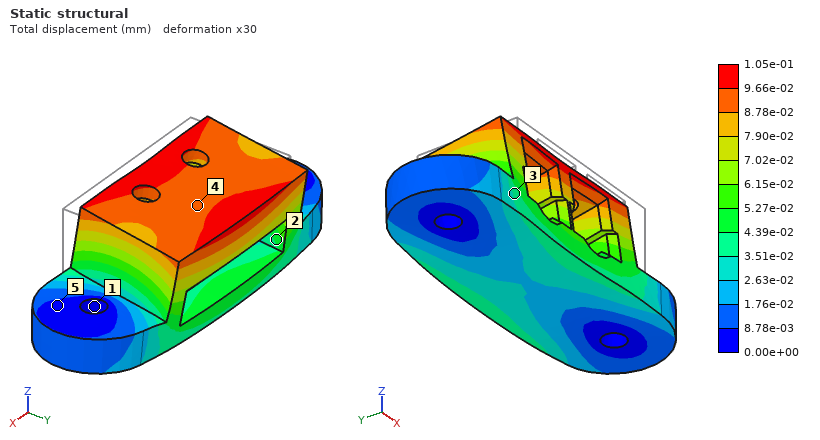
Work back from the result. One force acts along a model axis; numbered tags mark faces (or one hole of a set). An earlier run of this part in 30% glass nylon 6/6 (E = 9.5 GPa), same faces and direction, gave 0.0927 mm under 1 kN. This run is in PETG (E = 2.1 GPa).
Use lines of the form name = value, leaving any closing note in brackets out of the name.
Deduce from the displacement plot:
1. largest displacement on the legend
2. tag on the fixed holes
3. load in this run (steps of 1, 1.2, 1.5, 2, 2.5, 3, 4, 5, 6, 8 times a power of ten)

largest displacement on the legend = 1.05e-01 mm
tag on the fixed holes = 1
load in this run = 250 N
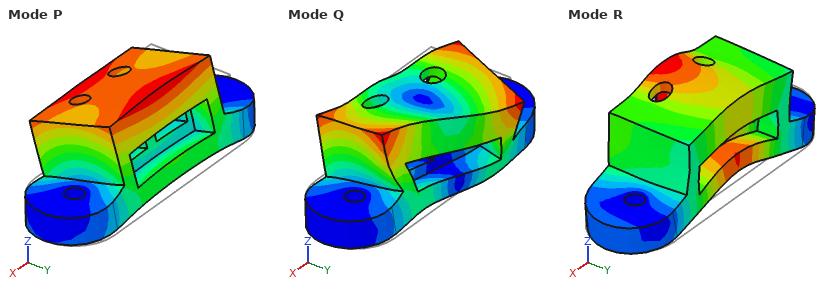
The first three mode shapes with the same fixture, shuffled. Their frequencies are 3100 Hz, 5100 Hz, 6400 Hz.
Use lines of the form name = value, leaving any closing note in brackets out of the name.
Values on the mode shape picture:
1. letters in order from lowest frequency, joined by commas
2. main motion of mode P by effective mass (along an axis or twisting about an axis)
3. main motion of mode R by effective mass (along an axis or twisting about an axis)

letters in order from lowest frequency, joined by commas = P, R, Q
main motion of mode P by effective mass = along Y
main motion of mode R by effective mass = along Z
